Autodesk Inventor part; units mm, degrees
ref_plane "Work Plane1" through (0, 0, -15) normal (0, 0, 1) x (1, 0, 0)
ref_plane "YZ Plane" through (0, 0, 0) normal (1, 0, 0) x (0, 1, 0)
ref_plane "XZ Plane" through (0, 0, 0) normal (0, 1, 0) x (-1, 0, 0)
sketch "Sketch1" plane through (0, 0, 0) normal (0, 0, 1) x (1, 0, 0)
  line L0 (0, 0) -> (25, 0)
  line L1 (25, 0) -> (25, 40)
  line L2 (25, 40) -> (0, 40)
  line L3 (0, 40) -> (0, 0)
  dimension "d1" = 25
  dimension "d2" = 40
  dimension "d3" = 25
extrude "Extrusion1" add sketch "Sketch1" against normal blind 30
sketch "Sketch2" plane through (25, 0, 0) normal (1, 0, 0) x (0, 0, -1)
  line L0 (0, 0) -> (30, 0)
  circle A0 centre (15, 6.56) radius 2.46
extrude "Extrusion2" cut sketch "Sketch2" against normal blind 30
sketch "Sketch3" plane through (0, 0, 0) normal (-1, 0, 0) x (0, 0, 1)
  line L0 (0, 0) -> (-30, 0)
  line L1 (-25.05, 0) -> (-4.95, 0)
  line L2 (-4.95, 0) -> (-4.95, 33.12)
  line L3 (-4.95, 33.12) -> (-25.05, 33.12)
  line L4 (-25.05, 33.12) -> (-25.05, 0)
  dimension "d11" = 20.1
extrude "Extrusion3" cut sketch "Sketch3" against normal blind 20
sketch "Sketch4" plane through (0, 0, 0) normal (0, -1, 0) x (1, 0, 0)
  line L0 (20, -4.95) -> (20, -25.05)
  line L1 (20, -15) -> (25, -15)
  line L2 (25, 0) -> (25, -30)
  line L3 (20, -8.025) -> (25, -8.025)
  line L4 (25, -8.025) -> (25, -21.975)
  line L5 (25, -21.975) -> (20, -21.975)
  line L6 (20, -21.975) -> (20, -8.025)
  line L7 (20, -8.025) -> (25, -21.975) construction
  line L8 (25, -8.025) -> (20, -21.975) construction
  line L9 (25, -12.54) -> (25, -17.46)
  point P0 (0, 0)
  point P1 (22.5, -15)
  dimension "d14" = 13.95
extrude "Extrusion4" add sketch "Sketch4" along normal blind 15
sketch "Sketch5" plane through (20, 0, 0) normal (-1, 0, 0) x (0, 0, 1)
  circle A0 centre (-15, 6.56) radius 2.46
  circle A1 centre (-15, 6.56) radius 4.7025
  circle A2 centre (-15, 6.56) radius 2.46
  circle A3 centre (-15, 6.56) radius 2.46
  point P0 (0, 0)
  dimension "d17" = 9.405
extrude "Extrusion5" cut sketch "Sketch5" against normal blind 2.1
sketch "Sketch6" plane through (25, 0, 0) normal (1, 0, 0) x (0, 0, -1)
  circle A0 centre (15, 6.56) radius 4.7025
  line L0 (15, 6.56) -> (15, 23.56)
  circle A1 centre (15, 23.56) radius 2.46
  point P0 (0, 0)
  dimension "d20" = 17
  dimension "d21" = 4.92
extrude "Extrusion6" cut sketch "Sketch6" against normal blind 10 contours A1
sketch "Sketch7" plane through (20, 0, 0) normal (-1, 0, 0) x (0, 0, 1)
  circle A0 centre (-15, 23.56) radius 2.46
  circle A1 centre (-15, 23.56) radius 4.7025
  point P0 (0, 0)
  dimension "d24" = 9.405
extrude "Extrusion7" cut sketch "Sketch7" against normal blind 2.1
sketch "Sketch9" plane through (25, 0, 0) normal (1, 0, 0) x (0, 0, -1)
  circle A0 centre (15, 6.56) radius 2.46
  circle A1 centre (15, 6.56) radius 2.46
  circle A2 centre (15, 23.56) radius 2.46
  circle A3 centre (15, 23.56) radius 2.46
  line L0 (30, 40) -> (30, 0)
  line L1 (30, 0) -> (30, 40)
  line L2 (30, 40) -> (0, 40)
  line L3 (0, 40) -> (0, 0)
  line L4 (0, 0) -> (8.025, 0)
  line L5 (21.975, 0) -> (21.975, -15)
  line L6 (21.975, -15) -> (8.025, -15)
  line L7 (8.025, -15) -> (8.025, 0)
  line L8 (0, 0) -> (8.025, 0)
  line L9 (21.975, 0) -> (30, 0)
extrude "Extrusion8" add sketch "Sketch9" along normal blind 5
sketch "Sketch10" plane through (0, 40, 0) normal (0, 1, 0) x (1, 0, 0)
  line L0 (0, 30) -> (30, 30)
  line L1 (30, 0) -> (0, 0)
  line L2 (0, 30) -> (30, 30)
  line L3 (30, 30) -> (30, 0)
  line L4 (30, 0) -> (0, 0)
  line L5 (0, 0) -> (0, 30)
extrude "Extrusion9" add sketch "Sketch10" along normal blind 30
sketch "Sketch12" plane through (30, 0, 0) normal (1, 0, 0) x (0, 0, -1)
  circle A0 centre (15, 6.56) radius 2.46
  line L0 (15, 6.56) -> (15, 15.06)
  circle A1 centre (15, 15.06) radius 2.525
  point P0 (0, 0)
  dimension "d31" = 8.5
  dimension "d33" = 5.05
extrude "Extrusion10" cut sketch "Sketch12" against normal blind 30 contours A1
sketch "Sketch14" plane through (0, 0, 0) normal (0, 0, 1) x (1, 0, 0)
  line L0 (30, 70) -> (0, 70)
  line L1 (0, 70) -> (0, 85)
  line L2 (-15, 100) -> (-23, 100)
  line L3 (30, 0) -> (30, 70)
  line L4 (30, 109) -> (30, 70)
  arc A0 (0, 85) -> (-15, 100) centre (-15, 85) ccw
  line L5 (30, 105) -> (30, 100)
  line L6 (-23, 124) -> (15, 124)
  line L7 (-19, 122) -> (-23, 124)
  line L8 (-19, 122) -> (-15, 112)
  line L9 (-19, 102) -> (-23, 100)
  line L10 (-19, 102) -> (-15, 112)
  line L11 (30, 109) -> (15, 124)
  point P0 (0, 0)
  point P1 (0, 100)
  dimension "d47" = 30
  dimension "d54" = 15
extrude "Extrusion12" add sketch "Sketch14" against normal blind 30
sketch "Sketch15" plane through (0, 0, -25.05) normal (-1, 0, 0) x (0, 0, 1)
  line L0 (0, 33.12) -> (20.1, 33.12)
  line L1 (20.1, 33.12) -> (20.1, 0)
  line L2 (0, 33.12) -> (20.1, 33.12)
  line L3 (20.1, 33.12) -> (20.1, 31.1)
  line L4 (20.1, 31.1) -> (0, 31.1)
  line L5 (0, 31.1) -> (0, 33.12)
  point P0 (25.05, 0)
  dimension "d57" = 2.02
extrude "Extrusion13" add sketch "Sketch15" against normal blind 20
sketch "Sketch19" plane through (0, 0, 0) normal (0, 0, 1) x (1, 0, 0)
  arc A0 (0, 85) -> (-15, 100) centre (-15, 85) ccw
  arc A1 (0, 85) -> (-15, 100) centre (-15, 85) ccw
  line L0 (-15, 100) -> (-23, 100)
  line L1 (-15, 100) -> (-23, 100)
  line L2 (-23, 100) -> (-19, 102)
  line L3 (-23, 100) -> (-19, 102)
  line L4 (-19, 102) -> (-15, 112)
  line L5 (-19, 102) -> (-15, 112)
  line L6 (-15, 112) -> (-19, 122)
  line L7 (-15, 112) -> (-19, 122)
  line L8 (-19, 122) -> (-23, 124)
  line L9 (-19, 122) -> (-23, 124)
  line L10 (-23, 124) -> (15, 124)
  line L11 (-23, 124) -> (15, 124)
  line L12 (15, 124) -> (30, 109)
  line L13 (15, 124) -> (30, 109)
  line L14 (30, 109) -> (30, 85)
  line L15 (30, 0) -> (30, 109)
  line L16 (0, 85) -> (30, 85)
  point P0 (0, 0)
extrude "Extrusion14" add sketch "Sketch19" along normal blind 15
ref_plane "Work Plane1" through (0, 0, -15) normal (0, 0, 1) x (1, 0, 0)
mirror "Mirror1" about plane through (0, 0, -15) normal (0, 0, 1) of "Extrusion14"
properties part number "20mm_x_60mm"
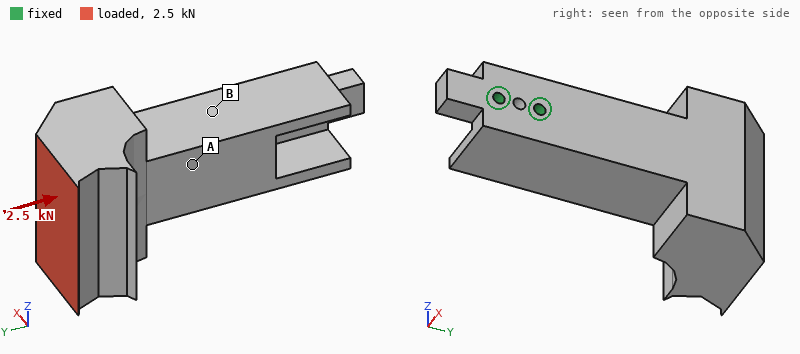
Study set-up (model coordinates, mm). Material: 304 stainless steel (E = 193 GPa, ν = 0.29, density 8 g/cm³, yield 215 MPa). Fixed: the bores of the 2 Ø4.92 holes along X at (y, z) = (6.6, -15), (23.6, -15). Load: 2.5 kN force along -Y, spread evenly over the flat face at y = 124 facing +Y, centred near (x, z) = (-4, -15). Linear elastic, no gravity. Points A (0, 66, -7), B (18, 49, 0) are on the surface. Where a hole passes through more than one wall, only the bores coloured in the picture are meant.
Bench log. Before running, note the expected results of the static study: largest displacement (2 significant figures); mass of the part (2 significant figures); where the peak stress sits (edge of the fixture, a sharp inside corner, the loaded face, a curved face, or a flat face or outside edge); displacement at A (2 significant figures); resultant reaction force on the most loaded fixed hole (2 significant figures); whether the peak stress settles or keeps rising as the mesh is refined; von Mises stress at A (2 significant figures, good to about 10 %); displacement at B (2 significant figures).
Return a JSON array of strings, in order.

["83 µm", "1.3 kg", "edge of the fixture", "32 µm", "3.4 kN", "keeps rising", "13 MPa", "16 µm"]
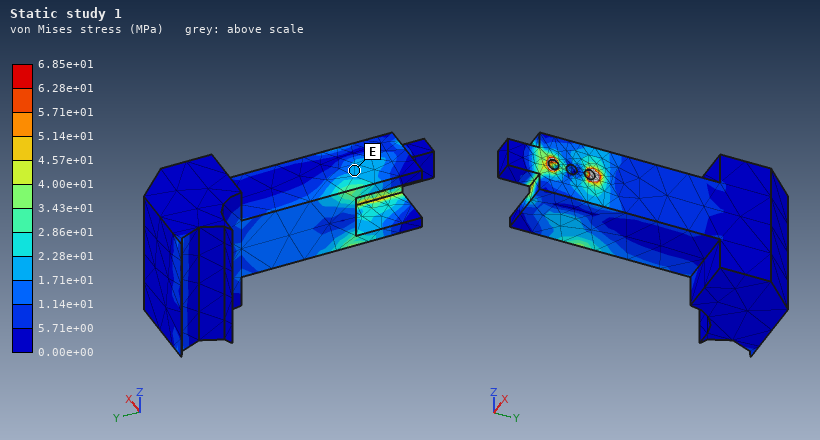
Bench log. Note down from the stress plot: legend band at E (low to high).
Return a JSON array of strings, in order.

["1.71e+01 to 2.28e+01 MPa"]
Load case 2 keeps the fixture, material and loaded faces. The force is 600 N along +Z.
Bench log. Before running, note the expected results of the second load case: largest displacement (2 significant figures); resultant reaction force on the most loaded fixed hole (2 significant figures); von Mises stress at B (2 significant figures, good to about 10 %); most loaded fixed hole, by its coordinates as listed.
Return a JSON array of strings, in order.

["58 µm", "3.2 kN", "11 MPa", "(23.6, -15)"]
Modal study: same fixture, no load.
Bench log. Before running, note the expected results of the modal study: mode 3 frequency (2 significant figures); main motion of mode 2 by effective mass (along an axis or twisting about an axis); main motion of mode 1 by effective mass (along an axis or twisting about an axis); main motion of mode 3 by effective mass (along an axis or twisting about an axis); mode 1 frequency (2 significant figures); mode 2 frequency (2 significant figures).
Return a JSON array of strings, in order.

["1700 Hz", "along Z", "along X", "twisting about Y", "670 Hz", "770 Hz"]
